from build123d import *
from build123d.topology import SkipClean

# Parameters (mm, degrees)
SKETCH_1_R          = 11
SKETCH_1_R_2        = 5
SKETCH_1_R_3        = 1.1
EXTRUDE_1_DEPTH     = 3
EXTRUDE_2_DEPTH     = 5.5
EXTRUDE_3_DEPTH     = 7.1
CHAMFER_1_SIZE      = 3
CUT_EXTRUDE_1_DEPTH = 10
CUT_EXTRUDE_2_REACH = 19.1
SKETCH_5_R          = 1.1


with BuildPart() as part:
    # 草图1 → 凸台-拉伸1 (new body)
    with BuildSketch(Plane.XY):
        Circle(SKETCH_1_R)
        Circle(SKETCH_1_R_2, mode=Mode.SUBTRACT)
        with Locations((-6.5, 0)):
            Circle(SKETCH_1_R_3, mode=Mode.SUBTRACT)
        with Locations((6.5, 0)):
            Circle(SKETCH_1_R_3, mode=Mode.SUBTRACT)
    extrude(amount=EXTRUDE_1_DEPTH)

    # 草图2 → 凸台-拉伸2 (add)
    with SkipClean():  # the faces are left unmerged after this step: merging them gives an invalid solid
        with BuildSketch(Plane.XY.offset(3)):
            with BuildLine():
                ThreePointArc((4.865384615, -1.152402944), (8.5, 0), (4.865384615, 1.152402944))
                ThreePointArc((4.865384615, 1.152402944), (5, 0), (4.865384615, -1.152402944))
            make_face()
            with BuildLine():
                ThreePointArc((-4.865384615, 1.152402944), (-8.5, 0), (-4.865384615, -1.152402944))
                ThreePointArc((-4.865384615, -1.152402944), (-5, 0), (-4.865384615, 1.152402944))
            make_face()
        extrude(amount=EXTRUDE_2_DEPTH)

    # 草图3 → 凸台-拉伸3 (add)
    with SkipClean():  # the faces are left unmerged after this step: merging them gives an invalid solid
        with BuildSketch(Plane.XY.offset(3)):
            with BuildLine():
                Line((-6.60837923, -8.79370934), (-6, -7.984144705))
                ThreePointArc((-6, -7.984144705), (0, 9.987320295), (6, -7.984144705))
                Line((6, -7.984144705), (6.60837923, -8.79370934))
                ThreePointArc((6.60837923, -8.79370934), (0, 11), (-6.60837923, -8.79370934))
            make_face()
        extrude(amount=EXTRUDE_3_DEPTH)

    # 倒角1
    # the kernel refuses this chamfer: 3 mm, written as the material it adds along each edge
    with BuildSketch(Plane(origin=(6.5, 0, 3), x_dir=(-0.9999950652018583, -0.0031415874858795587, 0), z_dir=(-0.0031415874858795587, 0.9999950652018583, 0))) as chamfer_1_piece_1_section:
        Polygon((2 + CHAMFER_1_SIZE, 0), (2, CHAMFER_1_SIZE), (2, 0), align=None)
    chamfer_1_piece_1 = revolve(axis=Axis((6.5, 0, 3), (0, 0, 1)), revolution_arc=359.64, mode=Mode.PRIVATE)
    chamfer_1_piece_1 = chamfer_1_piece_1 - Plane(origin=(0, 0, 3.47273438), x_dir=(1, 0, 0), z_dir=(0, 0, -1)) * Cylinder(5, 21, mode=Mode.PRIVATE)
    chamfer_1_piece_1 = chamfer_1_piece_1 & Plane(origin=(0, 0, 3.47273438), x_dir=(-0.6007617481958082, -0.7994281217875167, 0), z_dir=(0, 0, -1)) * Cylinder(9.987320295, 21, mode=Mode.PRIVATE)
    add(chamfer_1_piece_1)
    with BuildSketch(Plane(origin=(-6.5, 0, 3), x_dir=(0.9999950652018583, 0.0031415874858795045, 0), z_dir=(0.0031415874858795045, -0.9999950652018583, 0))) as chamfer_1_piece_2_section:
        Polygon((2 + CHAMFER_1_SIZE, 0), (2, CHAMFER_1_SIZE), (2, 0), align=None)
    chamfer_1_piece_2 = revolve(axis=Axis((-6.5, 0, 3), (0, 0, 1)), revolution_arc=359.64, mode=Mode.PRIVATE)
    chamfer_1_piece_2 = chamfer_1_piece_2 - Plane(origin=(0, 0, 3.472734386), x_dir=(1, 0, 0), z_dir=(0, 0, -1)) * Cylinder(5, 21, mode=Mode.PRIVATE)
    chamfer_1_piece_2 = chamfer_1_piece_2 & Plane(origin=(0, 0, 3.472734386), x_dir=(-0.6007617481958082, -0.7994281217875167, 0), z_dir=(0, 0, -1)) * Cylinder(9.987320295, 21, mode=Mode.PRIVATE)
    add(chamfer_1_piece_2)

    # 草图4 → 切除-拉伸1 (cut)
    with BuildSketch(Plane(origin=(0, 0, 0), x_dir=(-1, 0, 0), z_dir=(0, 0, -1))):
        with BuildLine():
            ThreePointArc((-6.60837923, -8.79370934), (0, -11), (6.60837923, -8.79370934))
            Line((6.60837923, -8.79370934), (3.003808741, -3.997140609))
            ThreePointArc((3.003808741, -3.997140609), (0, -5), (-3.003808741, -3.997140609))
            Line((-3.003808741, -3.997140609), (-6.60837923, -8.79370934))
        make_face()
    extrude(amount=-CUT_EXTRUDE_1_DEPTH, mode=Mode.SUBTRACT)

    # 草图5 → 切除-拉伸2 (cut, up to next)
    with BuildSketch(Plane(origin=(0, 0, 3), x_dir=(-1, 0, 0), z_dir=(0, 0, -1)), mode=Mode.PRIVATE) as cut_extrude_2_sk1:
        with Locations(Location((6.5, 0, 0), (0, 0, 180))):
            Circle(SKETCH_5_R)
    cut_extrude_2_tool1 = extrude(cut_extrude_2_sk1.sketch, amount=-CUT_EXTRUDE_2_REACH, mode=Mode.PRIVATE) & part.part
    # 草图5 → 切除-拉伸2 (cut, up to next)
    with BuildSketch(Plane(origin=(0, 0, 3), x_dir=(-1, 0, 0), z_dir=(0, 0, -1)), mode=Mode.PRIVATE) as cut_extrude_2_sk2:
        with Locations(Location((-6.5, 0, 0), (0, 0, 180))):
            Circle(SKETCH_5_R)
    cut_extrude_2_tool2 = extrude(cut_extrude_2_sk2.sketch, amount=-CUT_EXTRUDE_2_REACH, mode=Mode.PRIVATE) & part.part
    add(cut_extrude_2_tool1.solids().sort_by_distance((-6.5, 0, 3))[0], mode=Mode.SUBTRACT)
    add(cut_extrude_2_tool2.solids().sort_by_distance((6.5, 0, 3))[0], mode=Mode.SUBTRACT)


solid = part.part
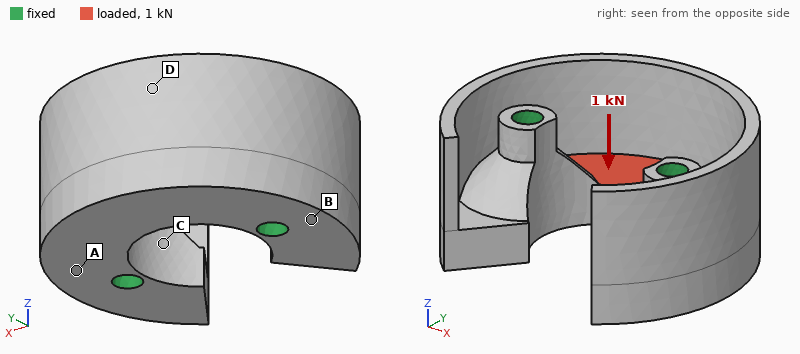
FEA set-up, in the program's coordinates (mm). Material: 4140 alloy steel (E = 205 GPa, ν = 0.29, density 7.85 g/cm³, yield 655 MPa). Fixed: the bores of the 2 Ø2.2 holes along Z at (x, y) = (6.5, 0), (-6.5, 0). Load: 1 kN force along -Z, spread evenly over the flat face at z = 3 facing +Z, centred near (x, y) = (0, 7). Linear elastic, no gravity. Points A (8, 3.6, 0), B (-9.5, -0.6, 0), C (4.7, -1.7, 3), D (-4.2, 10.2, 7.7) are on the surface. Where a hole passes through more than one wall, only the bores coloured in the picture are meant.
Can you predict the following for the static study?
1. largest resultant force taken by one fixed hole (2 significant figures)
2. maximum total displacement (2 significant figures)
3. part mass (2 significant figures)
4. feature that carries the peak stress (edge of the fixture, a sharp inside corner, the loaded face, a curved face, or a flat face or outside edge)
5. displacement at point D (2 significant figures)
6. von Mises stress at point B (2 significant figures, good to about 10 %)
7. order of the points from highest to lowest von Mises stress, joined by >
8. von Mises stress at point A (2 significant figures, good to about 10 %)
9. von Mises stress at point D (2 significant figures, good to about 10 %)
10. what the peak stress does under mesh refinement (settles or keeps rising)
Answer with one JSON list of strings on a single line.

["500 N", "19 µm", "10 g", "edge of the fixture", "13 µm", "31 MPa", "A > D > B > C", "67 MPa", "43 MPa", "keeps rising"]
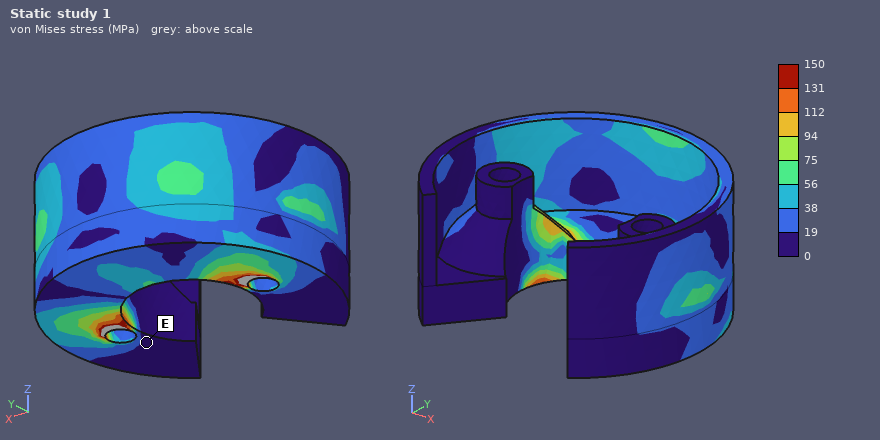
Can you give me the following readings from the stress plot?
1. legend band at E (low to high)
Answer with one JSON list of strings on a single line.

["0 to 19 MPa"]
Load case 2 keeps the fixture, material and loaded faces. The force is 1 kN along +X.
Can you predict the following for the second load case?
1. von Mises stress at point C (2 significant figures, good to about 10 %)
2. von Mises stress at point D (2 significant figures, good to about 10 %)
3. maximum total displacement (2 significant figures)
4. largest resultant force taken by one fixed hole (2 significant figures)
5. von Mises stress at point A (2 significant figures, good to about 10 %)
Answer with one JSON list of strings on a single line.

["13 MPa", "12 MPa", "5.8 µm", "560 N", "25 MPa"]
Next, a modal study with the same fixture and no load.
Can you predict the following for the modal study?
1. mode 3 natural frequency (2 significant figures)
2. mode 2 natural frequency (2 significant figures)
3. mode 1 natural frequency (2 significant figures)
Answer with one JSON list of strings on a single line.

["23 kHz", "23 kHz", "21 kHz"]
